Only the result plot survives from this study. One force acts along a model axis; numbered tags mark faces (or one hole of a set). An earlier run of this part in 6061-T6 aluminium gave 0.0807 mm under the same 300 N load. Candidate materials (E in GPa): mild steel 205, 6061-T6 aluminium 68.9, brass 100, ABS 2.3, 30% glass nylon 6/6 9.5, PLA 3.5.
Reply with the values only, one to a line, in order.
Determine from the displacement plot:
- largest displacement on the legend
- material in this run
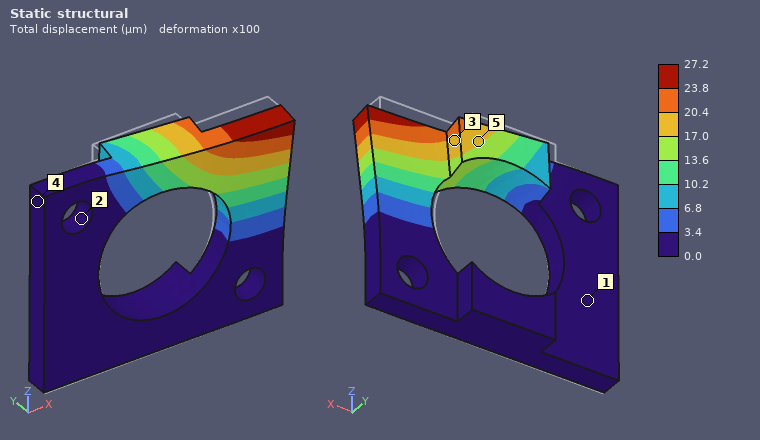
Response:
27.2 µm
mild steel
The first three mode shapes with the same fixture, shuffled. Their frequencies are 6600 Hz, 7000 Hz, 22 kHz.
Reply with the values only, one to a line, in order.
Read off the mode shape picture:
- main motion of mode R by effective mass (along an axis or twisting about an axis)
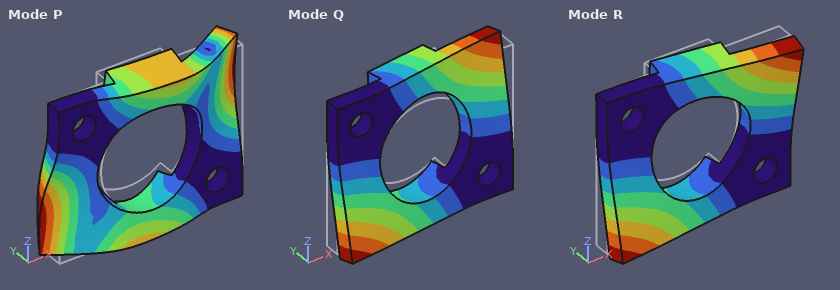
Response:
along Y
